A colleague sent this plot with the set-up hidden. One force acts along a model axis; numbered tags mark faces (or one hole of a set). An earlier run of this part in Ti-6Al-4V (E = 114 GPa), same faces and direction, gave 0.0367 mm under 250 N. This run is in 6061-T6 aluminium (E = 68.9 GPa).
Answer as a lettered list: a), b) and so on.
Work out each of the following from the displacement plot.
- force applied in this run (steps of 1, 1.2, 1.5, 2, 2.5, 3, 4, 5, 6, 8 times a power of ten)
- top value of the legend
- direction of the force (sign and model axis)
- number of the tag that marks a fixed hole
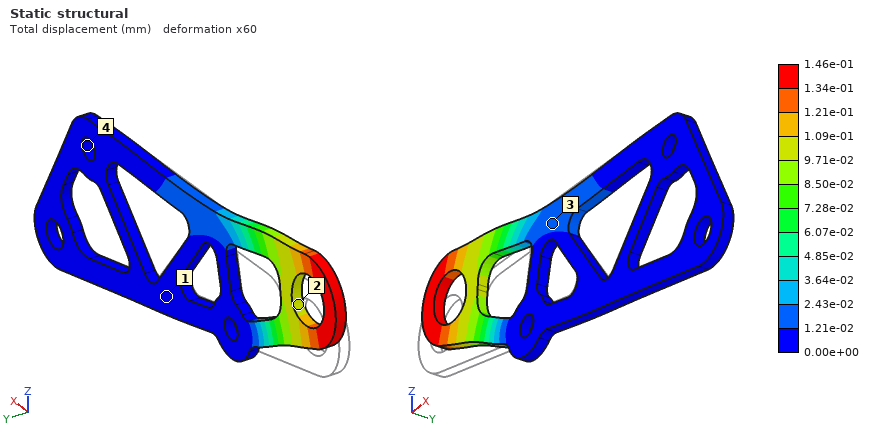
a) 600 N
b) 1.46e-01 mm
c) +Z
d) 4
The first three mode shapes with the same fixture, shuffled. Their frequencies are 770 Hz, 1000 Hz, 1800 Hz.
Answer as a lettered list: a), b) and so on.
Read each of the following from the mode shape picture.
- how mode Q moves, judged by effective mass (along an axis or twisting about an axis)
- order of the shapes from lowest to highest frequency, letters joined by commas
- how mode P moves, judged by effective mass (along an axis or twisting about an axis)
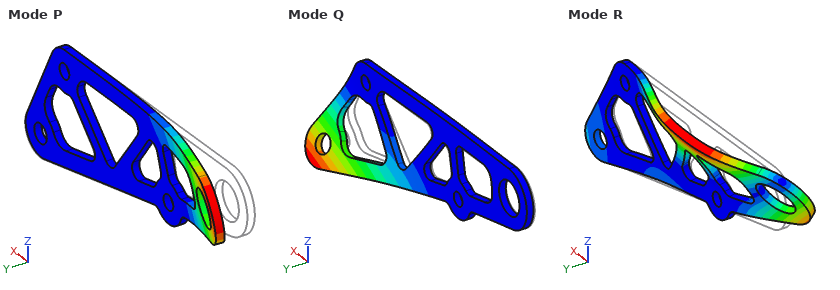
a) along Y
b) P, Q, R
c) along Y
